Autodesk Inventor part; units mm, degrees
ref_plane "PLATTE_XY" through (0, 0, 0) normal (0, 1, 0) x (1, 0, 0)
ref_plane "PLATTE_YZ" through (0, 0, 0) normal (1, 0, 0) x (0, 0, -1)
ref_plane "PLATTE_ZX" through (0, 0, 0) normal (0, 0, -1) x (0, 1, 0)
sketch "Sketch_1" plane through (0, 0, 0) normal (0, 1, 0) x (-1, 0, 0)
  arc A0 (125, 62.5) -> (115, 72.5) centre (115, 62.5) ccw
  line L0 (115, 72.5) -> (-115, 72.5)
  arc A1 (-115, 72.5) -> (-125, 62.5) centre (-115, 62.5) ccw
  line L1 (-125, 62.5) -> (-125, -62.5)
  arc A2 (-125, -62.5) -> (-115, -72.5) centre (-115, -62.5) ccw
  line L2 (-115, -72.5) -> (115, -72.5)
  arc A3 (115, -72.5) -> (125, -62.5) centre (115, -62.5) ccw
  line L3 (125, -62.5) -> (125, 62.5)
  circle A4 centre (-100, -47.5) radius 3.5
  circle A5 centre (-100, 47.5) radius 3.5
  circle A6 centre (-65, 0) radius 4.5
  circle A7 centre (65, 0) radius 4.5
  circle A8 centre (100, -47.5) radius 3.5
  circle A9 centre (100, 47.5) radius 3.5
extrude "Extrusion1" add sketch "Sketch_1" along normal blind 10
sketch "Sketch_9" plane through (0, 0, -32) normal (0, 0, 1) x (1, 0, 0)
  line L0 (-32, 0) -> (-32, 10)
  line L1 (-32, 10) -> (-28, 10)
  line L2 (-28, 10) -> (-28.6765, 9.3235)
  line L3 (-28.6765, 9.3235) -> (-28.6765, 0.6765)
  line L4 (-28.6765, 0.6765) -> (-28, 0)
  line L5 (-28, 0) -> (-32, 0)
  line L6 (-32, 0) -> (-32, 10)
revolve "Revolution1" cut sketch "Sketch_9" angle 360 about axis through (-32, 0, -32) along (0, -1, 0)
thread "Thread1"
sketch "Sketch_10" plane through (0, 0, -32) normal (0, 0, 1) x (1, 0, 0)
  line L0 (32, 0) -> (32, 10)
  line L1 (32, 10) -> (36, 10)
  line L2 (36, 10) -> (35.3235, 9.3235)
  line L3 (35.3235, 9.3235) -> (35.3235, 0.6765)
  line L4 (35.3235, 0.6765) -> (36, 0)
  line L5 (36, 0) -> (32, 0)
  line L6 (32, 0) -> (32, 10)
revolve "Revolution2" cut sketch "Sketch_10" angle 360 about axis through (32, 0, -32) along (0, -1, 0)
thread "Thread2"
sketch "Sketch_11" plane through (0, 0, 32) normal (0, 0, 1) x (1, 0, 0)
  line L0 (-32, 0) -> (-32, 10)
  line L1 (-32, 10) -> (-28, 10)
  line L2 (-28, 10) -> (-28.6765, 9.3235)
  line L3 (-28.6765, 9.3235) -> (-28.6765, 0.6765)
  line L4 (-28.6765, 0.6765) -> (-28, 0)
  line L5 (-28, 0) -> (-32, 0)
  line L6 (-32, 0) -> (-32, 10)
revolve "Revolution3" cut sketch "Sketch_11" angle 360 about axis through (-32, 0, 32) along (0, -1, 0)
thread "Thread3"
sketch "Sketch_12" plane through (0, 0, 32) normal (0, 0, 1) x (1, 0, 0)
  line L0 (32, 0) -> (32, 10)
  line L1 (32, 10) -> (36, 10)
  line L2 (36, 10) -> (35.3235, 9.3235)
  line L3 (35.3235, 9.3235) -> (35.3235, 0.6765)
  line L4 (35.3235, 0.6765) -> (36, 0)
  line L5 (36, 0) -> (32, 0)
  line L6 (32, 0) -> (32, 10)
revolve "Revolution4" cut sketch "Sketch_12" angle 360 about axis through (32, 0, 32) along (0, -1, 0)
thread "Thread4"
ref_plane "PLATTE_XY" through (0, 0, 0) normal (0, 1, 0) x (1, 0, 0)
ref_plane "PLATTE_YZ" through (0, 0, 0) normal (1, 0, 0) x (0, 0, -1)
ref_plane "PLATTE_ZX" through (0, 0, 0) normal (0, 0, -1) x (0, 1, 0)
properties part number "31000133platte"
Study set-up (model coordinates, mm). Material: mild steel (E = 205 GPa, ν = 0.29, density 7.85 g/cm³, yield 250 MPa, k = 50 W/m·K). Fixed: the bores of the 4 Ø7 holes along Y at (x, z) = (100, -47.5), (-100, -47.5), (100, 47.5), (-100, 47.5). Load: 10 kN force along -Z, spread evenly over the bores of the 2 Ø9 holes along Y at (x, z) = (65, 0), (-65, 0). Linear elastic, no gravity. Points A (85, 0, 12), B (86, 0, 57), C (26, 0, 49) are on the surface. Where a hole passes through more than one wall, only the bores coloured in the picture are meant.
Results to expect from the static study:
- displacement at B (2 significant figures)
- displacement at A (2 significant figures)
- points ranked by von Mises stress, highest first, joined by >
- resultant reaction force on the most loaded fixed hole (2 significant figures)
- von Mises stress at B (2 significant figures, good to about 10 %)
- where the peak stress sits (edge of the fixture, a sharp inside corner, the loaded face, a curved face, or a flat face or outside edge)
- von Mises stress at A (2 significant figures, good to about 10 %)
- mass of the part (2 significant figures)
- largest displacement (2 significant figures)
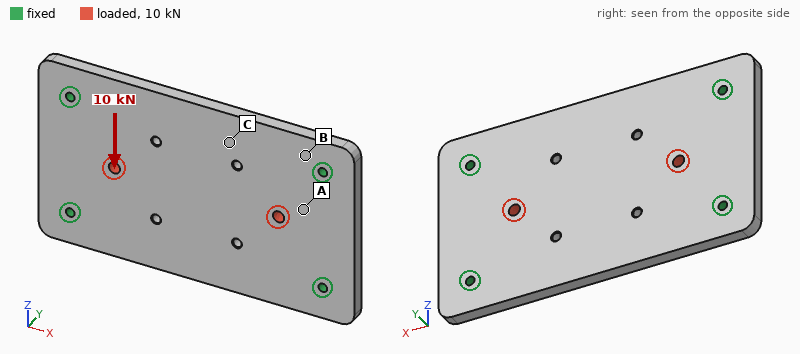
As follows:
1.1 µm
1.5 µm
A > B > C
2.8 kN
4.0 MPa
the loaded face
7.6 MPa
2.8 kg
3.6 µm
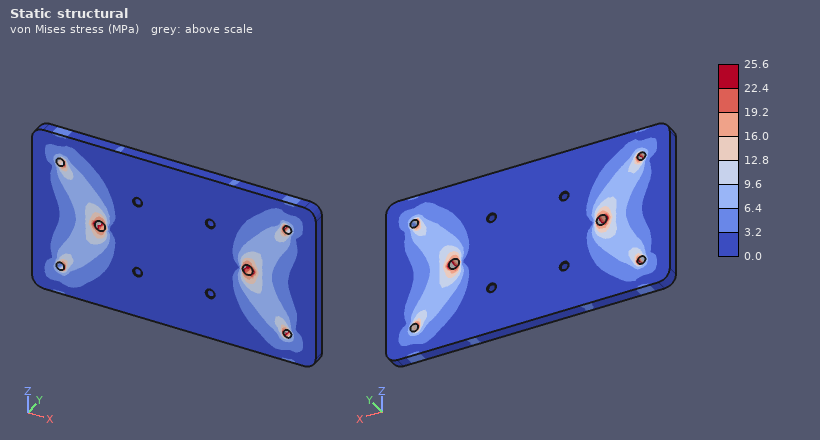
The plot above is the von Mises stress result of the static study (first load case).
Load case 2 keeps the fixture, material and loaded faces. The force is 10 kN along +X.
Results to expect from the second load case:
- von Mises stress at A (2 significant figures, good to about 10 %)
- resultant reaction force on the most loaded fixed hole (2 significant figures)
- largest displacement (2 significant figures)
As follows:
6.0 MPa
2.6 kN
3.0 µm
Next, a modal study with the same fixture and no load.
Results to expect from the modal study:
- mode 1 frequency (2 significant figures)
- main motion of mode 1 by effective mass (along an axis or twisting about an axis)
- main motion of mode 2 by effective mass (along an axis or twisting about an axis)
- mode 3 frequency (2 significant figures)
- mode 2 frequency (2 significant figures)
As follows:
1100 Hz
along Y
twisting about X
3000 Hz
1600 Hz
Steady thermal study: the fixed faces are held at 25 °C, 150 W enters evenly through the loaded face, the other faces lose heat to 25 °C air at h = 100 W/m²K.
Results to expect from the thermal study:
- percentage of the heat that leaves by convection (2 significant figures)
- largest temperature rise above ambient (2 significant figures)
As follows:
69 %
63 K
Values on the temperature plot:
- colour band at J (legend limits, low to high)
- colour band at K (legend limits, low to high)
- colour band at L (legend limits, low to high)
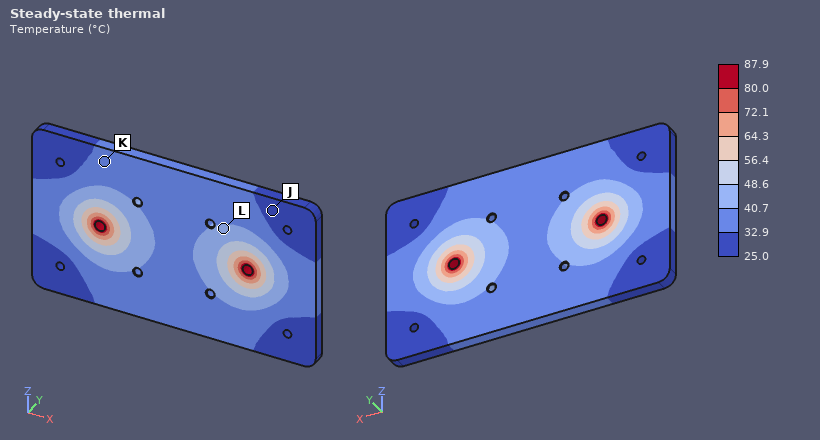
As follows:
25.0 to 32.9 °C
32.9 to 40.7 °C
40.7 to 48.6 °C
